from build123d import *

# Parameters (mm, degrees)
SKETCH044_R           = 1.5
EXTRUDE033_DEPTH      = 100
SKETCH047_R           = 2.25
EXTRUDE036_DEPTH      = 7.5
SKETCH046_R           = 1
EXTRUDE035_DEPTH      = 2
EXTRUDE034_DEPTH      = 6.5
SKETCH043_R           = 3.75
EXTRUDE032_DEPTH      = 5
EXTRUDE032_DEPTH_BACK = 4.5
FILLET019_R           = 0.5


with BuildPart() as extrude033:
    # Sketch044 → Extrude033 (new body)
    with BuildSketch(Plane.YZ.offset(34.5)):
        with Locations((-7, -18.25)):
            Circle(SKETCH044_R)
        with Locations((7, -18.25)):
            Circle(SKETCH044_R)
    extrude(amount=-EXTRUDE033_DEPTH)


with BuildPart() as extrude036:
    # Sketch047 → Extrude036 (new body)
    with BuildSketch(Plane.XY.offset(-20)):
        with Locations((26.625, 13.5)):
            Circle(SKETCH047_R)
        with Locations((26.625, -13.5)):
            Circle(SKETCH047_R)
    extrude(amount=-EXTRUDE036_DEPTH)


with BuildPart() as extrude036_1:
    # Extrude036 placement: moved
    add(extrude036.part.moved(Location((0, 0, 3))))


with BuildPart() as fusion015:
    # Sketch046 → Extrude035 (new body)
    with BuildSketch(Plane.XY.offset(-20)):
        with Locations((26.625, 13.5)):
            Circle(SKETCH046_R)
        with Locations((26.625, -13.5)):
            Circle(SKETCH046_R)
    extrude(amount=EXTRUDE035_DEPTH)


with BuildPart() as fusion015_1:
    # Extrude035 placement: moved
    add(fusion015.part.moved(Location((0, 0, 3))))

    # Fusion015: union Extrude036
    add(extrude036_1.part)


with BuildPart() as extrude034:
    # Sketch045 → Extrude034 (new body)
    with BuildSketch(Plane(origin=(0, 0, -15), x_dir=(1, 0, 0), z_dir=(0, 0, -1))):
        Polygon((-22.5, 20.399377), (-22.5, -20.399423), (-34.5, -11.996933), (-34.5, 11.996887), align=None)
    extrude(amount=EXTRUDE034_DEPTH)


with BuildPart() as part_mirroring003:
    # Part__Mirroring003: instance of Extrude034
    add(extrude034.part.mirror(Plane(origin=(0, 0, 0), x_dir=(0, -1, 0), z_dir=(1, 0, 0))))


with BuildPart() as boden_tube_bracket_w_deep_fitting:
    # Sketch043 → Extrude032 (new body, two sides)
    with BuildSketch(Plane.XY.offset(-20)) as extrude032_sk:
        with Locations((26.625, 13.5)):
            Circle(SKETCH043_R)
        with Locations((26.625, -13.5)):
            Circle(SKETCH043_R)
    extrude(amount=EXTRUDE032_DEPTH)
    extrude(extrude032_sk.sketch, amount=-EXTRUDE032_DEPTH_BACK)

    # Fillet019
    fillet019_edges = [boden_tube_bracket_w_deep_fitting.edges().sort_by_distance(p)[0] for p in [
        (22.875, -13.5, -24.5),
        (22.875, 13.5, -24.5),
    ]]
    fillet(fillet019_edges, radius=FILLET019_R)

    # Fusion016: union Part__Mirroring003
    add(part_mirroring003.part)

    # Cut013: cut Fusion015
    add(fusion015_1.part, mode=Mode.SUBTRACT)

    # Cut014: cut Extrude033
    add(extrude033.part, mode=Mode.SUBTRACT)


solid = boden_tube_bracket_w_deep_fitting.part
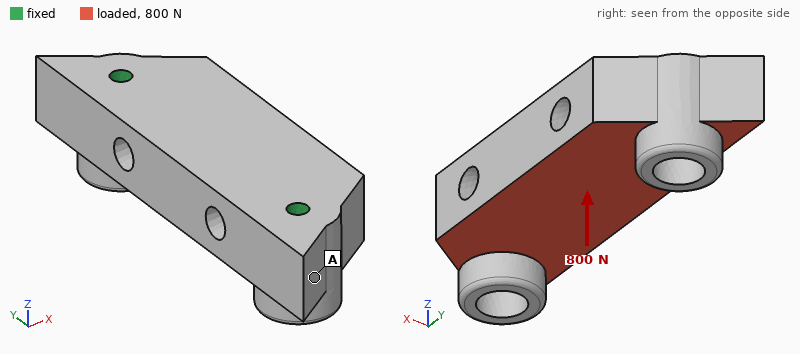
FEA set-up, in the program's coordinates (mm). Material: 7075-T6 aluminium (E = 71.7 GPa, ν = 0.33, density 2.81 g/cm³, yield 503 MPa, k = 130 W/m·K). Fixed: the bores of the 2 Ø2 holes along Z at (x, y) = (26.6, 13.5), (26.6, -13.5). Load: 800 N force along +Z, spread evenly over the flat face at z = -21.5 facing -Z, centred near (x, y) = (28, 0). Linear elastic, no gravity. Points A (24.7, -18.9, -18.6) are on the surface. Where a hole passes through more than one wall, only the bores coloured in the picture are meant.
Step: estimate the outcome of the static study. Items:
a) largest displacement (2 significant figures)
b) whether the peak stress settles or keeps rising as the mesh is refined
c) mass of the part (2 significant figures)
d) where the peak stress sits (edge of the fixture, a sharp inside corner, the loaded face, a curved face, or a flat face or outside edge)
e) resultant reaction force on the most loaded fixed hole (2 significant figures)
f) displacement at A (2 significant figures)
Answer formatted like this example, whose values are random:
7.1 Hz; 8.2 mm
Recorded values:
24 µm; keeps rising; 6.7 g; edge of the fixture; 470 N; 4.8 µm
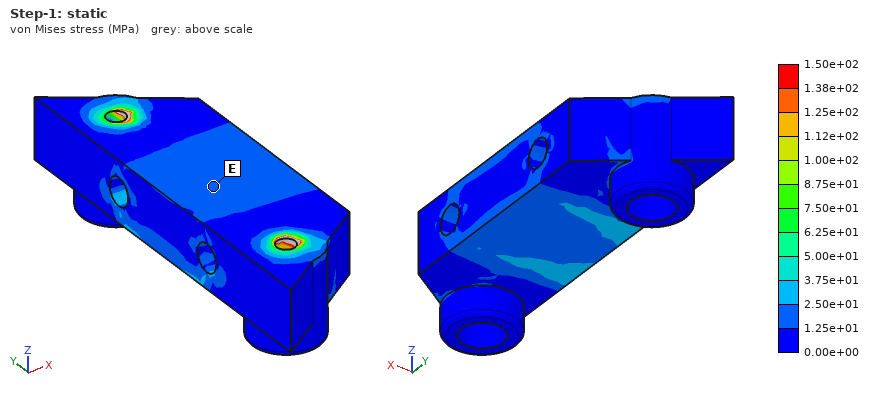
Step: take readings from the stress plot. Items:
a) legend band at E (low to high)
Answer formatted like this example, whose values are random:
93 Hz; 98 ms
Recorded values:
1.25e+01 to 2.50e+01 MPa
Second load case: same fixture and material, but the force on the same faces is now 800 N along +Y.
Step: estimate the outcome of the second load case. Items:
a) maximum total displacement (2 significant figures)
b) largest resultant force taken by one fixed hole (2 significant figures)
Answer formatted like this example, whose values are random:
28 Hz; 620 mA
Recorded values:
4.7 µm; 430 N
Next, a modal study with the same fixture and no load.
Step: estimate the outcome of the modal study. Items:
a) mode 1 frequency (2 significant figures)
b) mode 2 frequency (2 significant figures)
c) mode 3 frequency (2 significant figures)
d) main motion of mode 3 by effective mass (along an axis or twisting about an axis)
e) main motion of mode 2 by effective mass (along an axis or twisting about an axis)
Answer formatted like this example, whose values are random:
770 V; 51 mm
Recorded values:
12 kHz; 22 kHz; 30 kHz; along X; along Z
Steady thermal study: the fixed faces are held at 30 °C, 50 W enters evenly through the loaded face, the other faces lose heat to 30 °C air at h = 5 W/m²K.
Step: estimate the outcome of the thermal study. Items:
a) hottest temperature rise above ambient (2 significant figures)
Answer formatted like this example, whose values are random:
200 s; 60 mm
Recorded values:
45 K
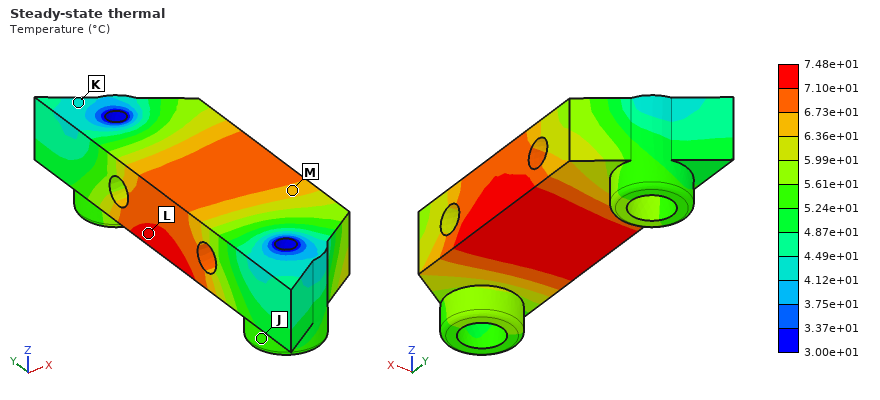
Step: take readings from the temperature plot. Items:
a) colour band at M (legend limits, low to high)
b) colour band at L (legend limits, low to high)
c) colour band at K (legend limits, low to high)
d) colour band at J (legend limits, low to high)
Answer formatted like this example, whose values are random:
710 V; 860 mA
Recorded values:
6.36e+01 to 6.73e+01 °C; 7.10e+01 to 7.48e+01 °C; 4.12e+01 to 4.49e+01 °C; 5.24e+01 to 5.61e+01 °C
